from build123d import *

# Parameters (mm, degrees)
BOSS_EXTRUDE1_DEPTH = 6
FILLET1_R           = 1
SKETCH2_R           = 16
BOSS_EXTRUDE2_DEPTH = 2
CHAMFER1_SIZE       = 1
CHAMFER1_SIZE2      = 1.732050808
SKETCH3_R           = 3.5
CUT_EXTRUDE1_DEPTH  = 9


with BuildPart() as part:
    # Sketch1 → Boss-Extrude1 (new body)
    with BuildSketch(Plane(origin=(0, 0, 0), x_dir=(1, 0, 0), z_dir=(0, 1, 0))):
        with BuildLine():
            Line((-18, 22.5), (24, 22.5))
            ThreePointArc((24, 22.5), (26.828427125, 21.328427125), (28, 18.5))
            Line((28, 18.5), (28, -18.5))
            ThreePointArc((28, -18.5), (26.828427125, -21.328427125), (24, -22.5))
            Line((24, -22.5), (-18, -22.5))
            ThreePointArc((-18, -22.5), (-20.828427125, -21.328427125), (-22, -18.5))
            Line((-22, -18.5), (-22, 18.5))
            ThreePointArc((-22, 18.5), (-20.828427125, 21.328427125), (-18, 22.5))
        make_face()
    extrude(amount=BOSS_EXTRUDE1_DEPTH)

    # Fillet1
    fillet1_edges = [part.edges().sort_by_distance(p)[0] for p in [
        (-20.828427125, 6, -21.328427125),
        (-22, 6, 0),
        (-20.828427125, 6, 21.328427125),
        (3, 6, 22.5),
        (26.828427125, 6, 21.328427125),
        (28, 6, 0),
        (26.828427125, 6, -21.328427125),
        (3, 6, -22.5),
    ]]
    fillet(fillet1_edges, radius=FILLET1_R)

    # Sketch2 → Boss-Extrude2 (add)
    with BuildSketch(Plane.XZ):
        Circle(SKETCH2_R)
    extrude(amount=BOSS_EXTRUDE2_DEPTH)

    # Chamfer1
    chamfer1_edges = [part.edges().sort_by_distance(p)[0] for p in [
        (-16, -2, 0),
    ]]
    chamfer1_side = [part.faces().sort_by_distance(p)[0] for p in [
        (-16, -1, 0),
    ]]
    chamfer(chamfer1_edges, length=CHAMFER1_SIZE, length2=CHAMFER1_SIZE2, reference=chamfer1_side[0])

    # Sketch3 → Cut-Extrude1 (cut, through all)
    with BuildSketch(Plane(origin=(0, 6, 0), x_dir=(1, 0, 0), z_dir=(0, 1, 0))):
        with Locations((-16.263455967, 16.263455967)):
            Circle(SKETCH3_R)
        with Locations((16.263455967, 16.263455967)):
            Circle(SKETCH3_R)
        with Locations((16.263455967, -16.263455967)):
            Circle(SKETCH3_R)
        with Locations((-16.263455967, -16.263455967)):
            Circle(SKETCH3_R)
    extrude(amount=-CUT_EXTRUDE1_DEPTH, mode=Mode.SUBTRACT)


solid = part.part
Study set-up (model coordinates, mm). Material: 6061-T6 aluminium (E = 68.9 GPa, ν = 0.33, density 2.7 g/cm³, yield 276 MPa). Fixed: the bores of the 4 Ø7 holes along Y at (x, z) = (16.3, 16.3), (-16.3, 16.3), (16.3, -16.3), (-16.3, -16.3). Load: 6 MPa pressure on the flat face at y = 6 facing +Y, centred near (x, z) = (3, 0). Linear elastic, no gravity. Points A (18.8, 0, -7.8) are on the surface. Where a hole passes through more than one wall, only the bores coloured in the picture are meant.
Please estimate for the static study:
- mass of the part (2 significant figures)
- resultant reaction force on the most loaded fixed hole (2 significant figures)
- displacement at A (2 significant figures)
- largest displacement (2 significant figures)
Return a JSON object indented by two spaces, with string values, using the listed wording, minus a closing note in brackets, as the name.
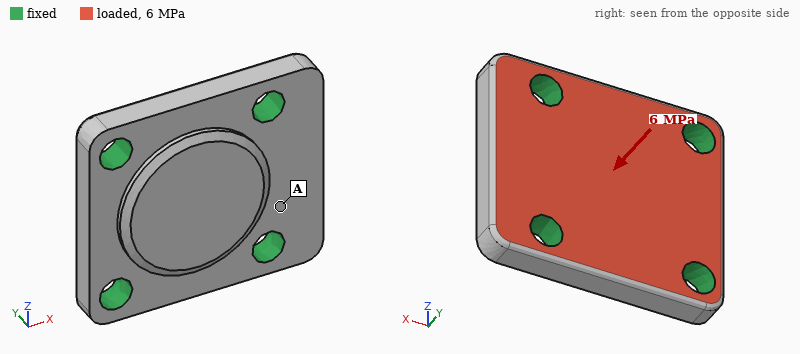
{
  "mass of the part": "38 g",
  "resultant reaction force on the most loaded fixed hole": "3.3 kN",
  "displacement at A": "9.2 µm",
  "largest displacement": "19 µm"
}
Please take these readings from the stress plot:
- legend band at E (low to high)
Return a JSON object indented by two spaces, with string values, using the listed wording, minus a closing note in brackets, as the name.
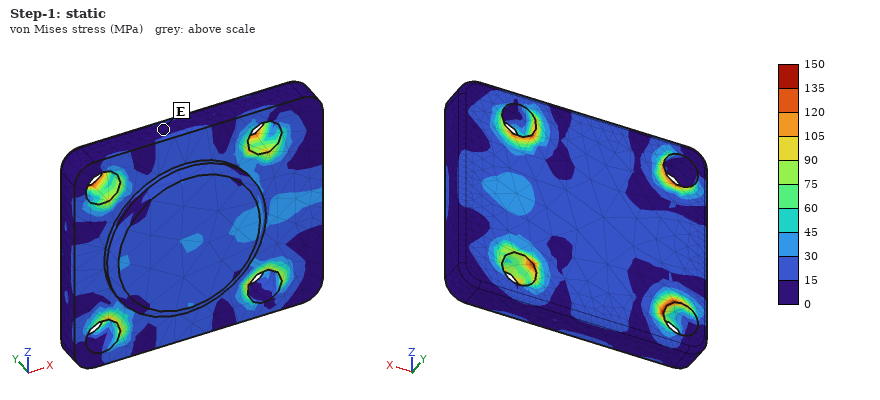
{
  "legend band at E": "0 to 15 MPa"
}
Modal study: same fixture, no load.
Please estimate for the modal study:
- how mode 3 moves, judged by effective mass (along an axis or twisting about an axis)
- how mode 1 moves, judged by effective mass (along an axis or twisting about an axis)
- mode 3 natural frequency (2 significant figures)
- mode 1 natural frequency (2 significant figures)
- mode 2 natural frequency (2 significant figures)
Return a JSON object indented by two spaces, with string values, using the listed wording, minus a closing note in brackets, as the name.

{
  "how mode 3 moves, judged by effective mass": "twisting about X",
  "how mode 1 moves, judged by effective mass": "along Y",
  "mode 3 natural frequency": "34 kHz",
  "mode 1 natural frequency": "23 kHz",
  "mode 2 natural frequency": "27 kHz"
}
